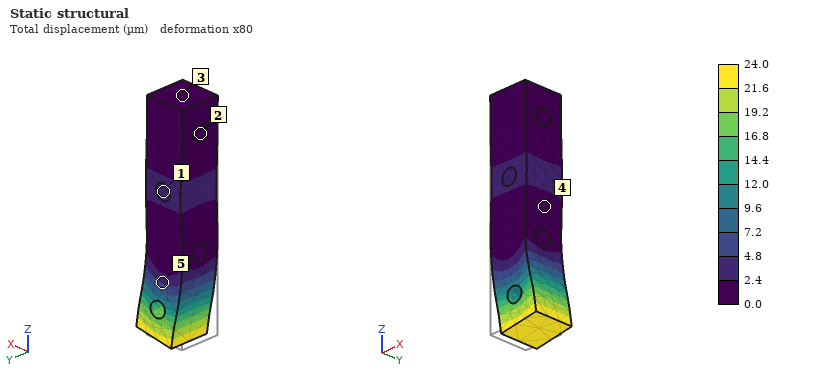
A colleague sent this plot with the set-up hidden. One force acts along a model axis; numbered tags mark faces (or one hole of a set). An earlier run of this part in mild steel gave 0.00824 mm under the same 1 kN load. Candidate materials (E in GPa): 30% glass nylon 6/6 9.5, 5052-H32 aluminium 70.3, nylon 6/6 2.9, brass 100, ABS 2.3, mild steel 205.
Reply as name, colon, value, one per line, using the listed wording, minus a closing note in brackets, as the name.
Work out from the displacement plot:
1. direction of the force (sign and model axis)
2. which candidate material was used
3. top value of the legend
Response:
direction of the force: +X
which candidate material was used: 5052-H32 aluminium
top value of the legend: 24.0 µm
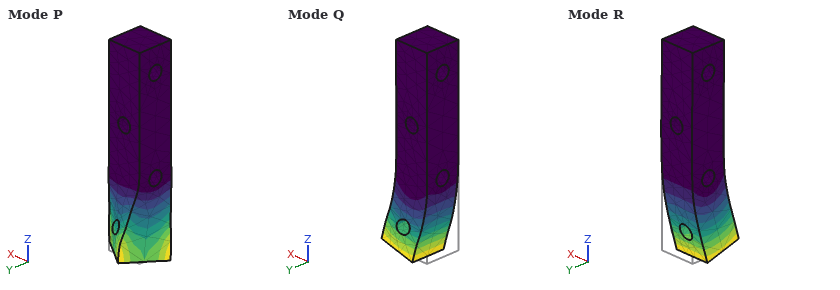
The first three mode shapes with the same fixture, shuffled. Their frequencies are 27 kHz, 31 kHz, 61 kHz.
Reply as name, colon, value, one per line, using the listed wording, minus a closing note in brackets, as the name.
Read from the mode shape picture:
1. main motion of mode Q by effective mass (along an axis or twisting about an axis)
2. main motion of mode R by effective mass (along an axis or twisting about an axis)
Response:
main motion of mode Q by effective mass: along X
main motion of mode R by effective mass: along Y
